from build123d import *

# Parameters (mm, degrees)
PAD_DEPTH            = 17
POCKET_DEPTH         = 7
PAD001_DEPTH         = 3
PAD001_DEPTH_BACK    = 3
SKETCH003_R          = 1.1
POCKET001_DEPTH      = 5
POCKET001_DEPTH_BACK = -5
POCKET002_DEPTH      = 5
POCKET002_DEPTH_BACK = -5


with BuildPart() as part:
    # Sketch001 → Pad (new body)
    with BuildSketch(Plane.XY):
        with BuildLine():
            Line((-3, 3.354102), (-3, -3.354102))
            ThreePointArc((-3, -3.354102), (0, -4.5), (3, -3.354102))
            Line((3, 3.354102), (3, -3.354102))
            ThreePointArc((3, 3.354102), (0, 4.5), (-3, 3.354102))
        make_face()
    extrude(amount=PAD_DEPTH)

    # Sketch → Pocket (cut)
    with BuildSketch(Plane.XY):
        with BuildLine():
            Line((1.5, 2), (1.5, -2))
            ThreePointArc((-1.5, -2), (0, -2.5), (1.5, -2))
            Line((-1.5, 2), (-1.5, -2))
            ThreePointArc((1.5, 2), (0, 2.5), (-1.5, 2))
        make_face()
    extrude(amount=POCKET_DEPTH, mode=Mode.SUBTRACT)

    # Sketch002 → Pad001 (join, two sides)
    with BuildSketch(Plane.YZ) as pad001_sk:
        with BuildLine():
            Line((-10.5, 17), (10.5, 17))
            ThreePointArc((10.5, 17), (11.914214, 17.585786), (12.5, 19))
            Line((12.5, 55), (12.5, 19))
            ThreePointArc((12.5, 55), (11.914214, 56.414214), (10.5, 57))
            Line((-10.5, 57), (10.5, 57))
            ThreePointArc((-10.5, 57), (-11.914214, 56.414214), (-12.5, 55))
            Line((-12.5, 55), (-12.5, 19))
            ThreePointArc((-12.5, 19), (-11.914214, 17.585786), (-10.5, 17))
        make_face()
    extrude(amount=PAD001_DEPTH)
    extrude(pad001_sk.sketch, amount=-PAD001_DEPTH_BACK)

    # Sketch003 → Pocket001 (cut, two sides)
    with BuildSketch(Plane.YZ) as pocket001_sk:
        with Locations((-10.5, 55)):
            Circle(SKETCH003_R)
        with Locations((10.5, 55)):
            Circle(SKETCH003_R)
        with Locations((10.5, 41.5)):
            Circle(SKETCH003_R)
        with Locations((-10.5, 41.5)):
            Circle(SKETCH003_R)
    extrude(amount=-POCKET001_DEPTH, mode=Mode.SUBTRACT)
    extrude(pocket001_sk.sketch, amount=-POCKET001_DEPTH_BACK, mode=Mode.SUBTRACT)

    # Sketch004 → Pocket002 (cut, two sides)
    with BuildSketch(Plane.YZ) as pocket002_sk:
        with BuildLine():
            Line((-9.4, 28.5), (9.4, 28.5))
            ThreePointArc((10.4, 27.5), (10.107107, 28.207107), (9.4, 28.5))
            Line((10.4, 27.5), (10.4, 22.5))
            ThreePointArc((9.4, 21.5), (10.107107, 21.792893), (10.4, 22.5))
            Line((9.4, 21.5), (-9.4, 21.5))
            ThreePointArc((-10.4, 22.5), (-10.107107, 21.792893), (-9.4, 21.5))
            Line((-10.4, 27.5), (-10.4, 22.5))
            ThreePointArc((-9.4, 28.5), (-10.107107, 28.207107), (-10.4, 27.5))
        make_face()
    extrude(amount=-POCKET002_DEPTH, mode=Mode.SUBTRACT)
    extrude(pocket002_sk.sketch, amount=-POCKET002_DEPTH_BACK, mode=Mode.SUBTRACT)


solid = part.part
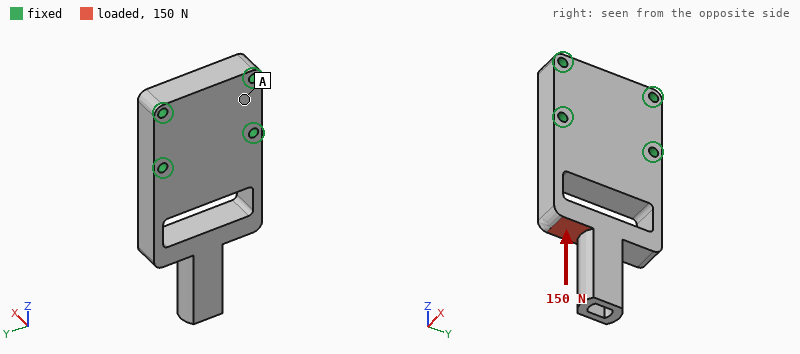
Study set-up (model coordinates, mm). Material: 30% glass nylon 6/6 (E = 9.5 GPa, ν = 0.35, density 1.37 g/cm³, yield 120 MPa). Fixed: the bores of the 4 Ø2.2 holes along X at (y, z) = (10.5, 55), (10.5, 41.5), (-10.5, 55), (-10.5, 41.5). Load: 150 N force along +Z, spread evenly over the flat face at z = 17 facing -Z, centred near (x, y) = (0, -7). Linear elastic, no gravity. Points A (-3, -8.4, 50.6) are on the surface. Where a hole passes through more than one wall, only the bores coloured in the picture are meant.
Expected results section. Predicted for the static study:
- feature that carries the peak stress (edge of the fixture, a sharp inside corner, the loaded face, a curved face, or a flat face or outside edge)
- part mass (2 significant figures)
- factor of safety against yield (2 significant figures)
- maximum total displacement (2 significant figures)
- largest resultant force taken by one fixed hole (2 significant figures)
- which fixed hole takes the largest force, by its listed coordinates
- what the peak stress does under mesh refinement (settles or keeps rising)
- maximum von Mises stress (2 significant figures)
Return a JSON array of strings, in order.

["a curved face", "7.9 g", "3.7", "48 µm", "120 N", "(-10.5, 41.5)", "settles", "32 MPa"]
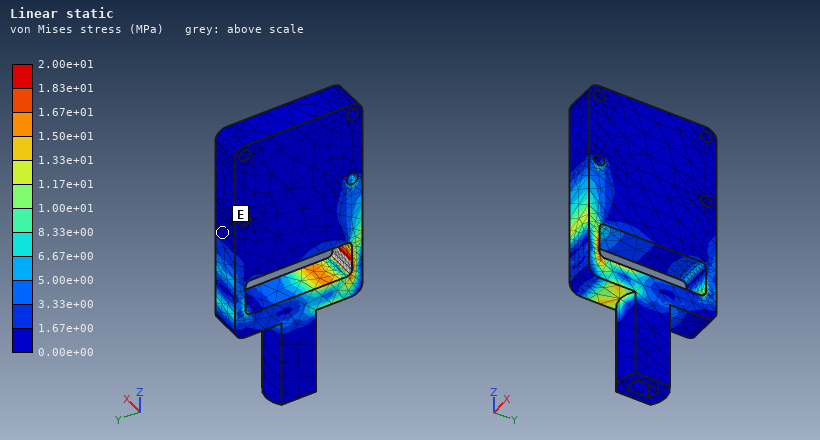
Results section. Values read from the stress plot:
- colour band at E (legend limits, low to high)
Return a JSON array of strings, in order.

["0.00e+00 to 1.67e+00 MPa"]
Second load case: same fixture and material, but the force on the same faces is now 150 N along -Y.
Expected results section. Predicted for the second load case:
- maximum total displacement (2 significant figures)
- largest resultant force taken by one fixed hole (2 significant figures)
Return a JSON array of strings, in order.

["0.15 mm", "180 N"]
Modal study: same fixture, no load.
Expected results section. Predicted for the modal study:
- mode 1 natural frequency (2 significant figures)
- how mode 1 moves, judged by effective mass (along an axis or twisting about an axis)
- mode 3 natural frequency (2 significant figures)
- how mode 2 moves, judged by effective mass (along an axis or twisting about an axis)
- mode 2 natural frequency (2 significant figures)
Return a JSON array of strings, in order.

["1500 Hz", "along X", "6100 Hz", "along Y", "3600 Hz"]
